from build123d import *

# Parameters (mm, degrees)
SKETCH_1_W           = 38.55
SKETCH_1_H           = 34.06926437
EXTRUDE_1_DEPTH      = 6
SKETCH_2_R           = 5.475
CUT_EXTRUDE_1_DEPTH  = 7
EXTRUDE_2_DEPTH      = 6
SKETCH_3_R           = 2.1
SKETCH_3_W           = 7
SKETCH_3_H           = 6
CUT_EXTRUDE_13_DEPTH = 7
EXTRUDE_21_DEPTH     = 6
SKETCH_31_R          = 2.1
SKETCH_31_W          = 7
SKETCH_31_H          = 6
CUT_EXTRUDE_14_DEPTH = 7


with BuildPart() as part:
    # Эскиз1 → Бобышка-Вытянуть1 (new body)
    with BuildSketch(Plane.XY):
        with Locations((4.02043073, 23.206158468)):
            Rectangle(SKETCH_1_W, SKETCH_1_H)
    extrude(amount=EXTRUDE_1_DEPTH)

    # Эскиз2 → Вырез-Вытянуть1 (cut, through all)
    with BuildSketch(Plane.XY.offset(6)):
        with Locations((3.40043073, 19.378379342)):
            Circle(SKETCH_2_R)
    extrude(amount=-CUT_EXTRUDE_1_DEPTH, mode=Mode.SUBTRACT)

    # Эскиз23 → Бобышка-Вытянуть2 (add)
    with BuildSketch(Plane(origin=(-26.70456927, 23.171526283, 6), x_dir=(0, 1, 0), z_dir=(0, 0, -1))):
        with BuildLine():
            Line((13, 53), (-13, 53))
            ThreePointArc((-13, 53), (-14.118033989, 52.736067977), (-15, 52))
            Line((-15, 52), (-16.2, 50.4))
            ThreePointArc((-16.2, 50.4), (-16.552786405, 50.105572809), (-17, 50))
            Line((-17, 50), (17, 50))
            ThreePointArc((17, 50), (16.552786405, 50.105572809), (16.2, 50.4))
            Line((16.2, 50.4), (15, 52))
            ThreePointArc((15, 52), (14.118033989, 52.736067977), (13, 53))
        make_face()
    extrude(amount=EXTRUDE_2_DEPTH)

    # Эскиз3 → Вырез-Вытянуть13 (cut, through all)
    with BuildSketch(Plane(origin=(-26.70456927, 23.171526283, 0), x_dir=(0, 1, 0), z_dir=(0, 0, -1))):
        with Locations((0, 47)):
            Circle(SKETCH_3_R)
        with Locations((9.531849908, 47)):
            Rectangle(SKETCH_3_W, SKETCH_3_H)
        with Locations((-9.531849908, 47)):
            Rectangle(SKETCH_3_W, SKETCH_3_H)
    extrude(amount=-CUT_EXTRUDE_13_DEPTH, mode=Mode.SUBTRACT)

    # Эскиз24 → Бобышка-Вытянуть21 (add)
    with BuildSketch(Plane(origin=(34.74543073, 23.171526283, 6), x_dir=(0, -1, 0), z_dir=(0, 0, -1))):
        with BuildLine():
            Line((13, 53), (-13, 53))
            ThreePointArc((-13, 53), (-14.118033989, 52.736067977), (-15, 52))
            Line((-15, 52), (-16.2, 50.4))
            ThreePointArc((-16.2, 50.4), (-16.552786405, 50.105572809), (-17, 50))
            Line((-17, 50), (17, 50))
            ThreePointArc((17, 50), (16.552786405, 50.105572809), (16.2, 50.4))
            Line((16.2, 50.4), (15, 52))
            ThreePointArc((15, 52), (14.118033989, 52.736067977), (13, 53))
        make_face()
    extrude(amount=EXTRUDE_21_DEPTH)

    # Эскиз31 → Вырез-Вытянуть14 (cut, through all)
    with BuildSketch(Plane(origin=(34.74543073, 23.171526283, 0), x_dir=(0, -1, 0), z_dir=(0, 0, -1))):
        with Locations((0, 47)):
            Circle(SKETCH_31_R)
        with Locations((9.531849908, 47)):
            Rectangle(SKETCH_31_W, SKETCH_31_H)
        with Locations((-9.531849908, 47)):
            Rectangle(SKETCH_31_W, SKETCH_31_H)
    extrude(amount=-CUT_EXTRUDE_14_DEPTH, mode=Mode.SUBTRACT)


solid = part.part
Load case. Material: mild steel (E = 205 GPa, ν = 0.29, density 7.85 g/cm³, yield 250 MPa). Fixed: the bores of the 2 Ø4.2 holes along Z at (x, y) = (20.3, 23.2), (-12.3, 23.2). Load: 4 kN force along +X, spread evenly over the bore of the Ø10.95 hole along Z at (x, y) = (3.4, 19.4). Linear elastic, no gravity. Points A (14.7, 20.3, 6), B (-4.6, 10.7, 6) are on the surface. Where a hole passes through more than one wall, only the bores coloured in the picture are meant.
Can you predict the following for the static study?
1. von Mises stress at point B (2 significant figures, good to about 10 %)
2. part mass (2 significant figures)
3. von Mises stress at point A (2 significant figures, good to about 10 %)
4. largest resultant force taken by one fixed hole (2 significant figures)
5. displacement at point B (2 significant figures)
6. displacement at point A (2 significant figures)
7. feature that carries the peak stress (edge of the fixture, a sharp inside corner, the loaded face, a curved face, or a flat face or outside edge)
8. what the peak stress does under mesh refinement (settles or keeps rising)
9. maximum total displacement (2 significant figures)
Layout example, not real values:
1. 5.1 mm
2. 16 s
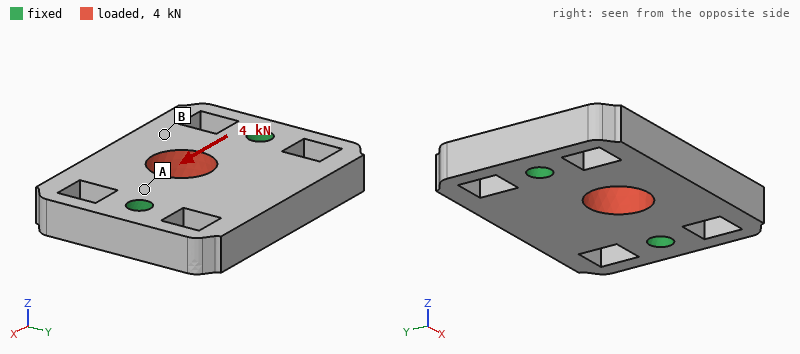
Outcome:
1. 7.7 MPa
2. 57 g
3. 33 MPa
4. 2.1 kN
5. 2.7 µm
6. 0.93 µm
7. edge of the fixture
8. keeps rising
9. 3.3 µm
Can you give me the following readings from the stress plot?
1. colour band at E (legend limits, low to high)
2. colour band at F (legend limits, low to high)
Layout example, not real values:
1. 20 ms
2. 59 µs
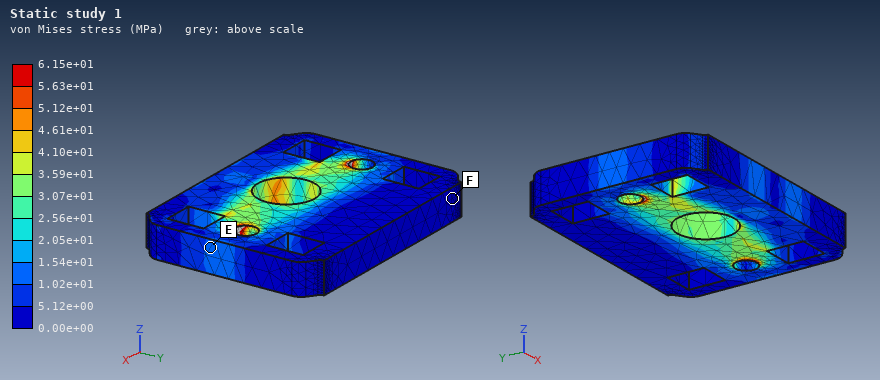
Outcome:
1. 1.02e+01 to 1.54e+01 MPa
2. 0.00e+00 to 5.12e+00 MPa
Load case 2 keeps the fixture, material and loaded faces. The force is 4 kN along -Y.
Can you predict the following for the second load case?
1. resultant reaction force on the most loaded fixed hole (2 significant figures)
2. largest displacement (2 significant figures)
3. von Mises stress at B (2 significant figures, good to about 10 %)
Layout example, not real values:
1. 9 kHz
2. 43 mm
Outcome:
1. 2.1 kN
2. 3.8 µm
3. 18 MPa
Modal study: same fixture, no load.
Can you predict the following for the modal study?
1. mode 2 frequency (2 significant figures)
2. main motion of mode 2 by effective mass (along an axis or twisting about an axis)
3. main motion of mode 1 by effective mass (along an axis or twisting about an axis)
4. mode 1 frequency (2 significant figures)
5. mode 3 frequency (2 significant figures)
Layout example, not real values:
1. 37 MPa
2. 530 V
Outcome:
1. 13 kHz
2. along Z
3. twisting about X
4. 10 kHz
5. 19 kHz
